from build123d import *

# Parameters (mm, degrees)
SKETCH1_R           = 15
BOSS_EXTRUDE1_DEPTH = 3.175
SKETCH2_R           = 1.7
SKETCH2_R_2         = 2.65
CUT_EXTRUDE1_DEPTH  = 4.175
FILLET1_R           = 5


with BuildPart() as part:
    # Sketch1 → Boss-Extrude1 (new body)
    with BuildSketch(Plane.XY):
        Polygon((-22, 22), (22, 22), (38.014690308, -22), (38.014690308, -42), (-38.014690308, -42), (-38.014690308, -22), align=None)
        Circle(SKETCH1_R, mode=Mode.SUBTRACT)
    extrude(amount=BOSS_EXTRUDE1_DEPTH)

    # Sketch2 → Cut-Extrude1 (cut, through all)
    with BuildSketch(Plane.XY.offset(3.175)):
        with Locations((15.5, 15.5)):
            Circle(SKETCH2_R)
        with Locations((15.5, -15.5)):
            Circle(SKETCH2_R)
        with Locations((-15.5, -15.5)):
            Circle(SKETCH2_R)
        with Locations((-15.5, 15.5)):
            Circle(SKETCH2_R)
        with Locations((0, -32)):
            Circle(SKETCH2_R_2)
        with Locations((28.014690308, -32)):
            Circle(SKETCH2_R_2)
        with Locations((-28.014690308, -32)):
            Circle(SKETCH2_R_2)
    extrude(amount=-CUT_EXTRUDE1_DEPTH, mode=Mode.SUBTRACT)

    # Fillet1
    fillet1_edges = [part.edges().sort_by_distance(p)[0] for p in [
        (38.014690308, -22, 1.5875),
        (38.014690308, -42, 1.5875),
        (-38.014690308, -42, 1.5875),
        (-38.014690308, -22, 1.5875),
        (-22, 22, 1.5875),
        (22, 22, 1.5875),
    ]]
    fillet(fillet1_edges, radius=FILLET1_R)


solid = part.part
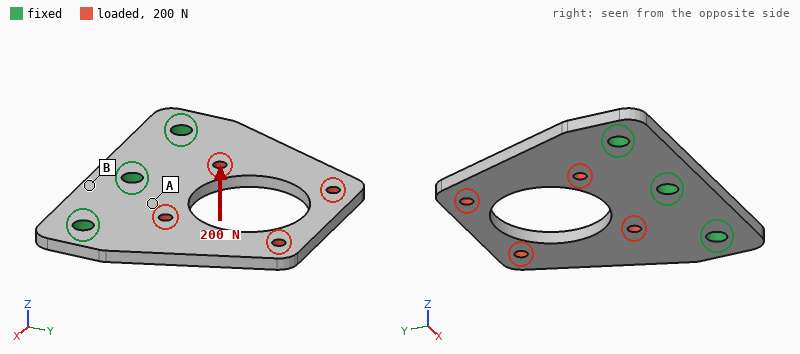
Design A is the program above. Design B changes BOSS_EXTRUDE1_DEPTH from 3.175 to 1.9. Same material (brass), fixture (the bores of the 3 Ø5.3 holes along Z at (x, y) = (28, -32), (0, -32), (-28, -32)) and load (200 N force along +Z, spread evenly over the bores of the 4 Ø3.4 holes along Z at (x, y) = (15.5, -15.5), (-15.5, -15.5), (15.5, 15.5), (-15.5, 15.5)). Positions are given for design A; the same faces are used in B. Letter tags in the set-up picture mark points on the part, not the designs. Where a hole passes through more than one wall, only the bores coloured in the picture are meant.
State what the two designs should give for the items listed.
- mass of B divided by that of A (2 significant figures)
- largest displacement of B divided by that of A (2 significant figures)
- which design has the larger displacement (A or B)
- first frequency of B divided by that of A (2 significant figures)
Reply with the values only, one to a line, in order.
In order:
0.60
4.5
B
0.61
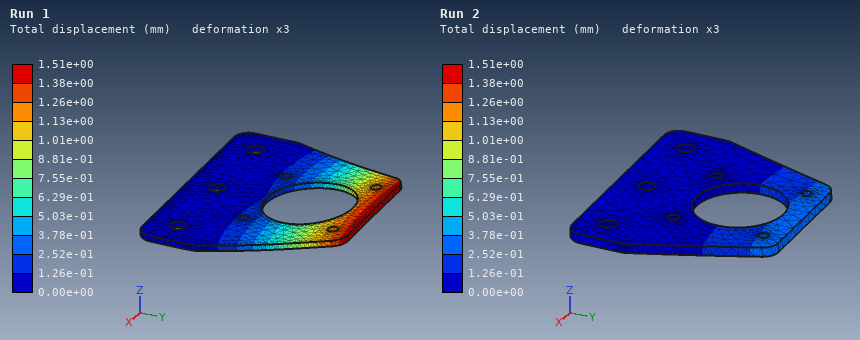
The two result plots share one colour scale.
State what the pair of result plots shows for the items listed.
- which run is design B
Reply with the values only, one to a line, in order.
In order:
Run 1
